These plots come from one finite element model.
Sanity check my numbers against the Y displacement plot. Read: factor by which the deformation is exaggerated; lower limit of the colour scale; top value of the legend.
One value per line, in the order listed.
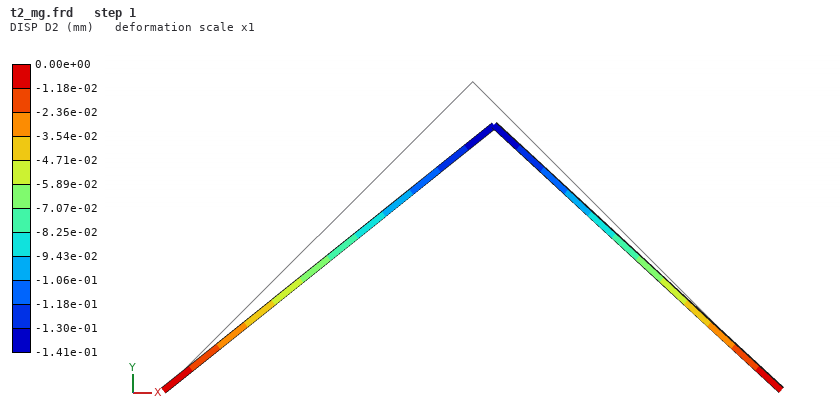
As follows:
1
-1.41e-01 mm
0.00e+00 mm
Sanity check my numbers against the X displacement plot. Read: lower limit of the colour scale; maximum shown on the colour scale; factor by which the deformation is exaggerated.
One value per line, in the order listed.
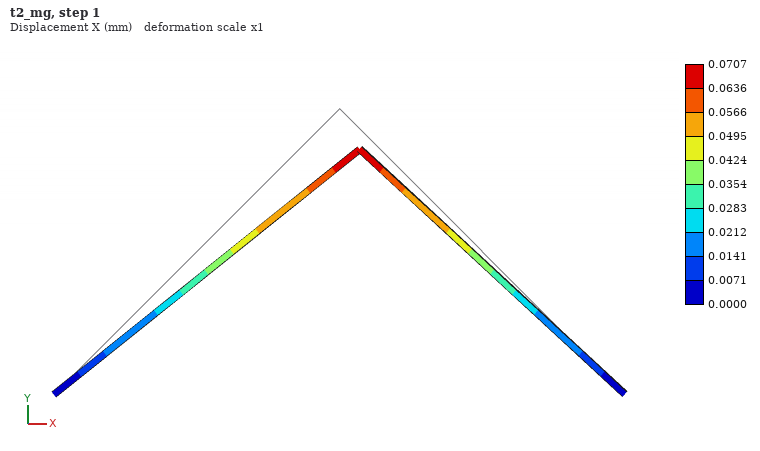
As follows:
0.0000 mm
0.0707 mm
1
